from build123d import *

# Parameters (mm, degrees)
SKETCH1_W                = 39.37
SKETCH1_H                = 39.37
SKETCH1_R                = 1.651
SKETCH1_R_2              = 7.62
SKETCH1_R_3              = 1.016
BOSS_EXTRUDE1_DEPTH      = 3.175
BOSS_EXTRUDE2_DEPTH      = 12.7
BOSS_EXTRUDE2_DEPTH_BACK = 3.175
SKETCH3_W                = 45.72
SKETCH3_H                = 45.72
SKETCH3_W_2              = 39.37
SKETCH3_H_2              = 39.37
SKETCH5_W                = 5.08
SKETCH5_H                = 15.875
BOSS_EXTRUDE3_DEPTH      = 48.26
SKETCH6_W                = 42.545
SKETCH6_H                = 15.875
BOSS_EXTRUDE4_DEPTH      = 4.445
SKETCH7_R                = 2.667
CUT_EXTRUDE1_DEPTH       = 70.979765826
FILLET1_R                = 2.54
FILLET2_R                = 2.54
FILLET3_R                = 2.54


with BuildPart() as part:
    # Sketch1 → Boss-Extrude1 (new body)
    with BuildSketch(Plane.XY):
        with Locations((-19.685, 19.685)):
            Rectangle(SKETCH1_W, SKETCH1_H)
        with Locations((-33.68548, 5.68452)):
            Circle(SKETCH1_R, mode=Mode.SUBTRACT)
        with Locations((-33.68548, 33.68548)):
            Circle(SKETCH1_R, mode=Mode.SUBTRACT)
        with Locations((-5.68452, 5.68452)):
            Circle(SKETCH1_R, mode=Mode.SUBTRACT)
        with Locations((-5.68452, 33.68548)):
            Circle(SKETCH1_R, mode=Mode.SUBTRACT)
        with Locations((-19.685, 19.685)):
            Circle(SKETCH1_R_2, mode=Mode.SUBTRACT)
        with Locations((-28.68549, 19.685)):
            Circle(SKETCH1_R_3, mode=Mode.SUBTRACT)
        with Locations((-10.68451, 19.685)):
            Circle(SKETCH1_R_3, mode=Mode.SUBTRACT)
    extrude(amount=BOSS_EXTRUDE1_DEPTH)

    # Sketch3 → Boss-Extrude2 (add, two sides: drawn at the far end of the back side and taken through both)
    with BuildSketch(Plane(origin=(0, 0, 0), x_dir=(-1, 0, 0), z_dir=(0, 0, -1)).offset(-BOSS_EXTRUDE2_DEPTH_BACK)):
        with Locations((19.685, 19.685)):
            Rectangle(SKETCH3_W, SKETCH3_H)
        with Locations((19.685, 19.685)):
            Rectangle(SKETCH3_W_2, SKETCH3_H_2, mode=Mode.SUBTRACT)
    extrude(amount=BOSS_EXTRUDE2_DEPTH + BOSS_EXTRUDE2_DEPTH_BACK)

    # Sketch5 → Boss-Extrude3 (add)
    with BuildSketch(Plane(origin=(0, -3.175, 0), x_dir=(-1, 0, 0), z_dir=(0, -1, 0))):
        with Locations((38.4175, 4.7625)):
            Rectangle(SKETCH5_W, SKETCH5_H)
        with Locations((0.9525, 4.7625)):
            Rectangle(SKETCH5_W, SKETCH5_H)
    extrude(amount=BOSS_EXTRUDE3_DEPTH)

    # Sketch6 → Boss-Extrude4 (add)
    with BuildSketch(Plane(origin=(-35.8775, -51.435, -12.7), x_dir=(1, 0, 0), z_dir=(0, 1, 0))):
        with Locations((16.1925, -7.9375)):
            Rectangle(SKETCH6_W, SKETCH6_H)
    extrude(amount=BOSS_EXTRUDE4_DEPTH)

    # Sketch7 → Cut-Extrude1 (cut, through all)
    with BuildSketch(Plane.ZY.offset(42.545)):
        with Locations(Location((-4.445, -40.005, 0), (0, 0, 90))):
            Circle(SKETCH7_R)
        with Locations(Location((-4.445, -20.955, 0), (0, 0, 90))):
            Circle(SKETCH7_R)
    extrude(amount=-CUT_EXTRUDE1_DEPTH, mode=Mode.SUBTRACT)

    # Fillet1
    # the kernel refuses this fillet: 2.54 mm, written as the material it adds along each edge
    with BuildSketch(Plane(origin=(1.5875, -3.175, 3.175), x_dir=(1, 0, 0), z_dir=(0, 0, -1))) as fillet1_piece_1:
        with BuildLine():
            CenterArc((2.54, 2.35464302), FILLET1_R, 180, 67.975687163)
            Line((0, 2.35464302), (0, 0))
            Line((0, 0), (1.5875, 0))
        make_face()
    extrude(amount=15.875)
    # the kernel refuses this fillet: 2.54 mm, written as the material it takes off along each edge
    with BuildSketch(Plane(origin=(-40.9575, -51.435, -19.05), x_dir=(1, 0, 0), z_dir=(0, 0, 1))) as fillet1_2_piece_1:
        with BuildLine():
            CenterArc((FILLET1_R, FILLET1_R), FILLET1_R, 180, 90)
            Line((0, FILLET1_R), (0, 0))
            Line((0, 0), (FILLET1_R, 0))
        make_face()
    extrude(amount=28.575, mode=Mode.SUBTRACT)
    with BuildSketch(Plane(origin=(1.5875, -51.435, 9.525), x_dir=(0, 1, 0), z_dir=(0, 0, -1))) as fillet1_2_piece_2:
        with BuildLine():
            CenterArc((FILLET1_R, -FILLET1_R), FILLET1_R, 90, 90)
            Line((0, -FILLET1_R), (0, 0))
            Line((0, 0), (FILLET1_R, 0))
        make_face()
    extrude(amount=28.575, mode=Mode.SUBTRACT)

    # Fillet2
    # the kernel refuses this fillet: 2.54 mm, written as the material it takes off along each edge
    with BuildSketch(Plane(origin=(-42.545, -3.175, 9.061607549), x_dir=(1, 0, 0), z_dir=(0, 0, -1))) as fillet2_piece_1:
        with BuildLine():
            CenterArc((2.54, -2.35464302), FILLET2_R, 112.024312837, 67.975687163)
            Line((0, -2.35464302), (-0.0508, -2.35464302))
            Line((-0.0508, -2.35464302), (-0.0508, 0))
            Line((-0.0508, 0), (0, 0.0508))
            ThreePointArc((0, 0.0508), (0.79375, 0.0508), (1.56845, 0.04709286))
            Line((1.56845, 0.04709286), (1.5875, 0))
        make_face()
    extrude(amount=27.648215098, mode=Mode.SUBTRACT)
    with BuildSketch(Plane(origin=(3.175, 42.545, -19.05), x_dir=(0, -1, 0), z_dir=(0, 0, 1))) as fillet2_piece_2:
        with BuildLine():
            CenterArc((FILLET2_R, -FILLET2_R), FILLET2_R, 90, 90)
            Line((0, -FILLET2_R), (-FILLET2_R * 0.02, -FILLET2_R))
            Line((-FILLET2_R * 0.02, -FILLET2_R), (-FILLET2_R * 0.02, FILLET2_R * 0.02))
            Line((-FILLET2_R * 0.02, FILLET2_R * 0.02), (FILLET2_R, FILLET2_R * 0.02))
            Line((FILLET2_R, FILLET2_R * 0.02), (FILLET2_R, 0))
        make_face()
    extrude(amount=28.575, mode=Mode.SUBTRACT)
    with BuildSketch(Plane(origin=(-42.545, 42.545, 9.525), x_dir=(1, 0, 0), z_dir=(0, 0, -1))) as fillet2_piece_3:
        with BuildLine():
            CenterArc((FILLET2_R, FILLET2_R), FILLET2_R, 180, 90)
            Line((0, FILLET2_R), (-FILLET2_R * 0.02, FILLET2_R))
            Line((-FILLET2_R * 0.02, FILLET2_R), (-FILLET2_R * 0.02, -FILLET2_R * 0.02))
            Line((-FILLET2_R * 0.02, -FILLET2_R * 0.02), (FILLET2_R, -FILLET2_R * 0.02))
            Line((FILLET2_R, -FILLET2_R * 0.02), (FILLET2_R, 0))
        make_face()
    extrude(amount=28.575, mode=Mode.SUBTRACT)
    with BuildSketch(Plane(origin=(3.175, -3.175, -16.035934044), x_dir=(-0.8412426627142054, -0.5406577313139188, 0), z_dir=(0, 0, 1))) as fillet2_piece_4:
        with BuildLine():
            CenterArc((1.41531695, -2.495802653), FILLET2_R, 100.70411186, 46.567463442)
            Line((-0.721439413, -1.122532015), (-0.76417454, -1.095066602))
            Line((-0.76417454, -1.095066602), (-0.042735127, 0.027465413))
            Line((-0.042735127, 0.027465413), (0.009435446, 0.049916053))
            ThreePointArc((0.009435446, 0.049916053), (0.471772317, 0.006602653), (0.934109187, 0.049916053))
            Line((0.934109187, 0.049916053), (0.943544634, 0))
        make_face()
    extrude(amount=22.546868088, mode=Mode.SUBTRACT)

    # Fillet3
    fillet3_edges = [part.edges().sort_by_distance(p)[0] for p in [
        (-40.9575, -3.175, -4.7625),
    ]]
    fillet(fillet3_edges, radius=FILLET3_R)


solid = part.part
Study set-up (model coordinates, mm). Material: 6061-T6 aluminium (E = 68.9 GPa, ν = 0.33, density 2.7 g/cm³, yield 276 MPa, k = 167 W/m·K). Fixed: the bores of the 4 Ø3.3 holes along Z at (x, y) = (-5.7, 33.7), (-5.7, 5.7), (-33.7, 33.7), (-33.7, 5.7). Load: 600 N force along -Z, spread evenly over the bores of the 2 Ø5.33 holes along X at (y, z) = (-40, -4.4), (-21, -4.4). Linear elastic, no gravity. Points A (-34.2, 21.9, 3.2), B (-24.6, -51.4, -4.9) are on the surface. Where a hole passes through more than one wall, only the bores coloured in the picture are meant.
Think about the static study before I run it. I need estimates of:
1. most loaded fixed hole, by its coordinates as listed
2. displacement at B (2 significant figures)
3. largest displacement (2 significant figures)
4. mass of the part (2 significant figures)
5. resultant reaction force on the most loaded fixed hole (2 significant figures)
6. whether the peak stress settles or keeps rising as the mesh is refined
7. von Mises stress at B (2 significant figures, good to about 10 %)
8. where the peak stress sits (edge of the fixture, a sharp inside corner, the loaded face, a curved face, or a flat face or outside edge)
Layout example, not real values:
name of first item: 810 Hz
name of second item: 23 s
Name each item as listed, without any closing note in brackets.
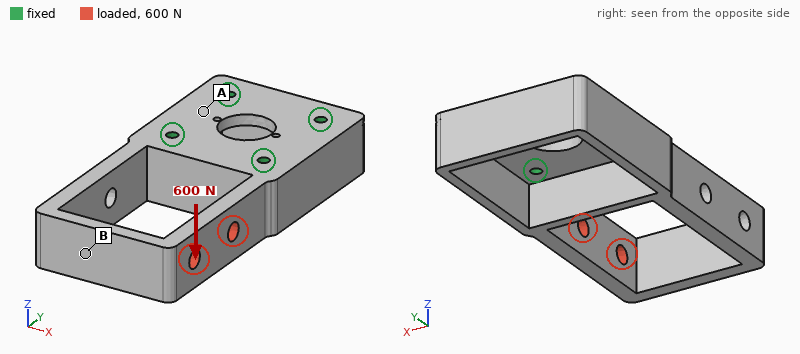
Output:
most loaded fixed hole, by its coordinates as listed: (-5.7, 5.7)
displacement at B: 0.14 mm
largest displacement: 0.28 mm
mass of the part: 60 g
resultant reaction force on the most loaded fixed hole: 1.3 kN
whether the peak stress settles or keeps rising as the mesh is refined: keeps rising
von Mises stress at B: 23 MPa
where the peak stress sits: edge of the fixture
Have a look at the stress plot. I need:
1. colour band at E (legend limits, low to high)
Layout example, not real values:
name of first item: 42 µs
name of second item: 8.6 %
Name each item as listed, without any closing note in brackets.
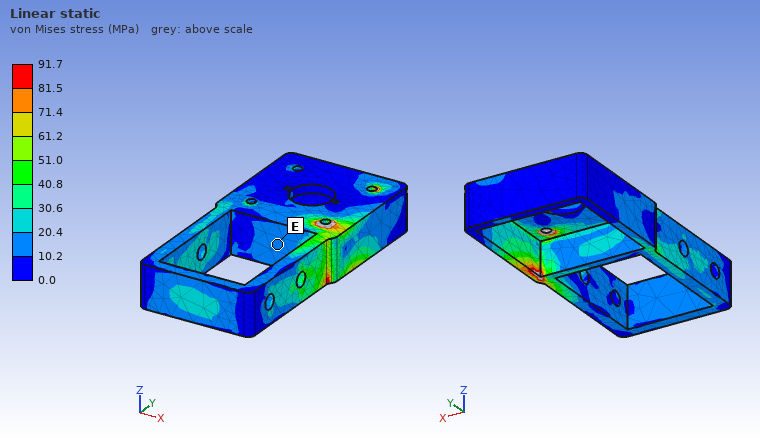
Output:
colour band at E: 10.2 to 20.4 MPa
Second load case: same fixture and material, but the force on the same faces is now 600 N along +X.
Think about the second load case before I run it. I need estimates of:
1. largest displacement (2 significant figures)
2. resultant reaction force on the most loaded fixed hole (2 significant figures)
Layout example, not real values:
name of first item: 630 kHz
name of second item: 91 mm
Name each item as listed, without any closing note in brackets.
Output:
largest displacement: 0.25 mm
resultant reaction force on the most loaded fixed hole: 500 N
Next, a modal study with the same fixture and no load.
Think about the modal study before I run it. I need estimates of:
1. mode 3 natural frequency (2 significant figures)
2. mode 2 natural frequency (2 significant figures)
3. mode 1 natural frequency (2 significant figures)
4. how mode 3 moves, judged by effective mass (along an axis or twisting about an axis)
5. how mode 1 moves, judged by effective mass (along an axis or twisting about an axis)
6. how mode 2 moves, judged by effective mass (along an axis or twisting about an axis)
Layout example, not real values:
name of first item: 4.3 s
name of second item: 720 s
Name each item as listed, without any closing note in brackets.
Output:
mode 3 natural frequency: 3000 Hz
mode 2 natural frequency: 2000 Hz
mode 1 natural frequency: 1700 Hz
how mode 3 moves, judged by effective mass: twisting about Y
how mode 1 moves, judged by effective mass: along X
how mode 2 moves, judged by effective mass: along Z
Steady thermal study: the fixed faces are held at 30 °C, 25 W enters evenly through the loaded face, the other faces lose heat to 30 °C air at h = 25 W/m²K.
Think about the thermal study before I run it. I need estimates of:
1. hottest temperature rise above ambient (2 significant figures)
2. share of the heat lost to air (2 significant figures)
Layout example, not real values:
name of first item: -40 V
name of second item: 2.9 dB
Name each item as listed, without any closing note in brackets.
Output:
hottest temperature rise above ambient: 47 K
share of the heat lost to air: 17 %
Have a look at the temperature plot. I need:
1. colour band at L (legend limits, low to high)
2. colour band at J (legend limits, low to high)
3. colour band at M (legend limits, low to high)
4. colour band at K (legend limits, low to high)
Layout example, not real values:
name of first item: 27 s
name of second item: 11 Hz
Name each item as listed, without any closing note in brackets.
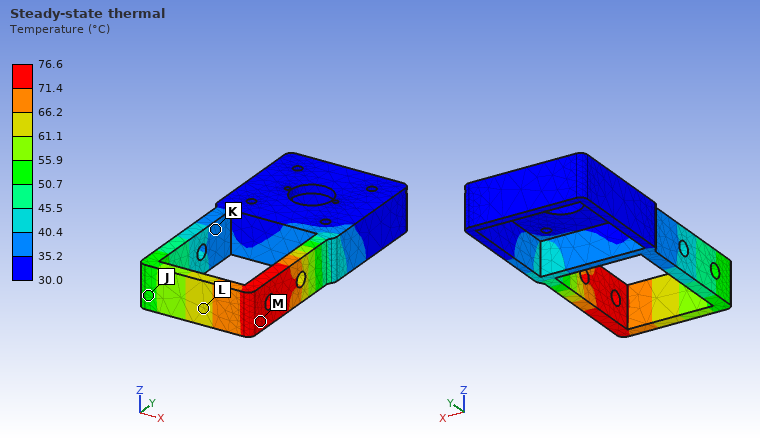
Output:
colour band at L: 61.1 to 66.2 °C
colour band at J: 50.7 to 55.9 °C
colour band at M: 71.4 to 76.6 °C
colour band at K: 35.2 to 40.4 °C
